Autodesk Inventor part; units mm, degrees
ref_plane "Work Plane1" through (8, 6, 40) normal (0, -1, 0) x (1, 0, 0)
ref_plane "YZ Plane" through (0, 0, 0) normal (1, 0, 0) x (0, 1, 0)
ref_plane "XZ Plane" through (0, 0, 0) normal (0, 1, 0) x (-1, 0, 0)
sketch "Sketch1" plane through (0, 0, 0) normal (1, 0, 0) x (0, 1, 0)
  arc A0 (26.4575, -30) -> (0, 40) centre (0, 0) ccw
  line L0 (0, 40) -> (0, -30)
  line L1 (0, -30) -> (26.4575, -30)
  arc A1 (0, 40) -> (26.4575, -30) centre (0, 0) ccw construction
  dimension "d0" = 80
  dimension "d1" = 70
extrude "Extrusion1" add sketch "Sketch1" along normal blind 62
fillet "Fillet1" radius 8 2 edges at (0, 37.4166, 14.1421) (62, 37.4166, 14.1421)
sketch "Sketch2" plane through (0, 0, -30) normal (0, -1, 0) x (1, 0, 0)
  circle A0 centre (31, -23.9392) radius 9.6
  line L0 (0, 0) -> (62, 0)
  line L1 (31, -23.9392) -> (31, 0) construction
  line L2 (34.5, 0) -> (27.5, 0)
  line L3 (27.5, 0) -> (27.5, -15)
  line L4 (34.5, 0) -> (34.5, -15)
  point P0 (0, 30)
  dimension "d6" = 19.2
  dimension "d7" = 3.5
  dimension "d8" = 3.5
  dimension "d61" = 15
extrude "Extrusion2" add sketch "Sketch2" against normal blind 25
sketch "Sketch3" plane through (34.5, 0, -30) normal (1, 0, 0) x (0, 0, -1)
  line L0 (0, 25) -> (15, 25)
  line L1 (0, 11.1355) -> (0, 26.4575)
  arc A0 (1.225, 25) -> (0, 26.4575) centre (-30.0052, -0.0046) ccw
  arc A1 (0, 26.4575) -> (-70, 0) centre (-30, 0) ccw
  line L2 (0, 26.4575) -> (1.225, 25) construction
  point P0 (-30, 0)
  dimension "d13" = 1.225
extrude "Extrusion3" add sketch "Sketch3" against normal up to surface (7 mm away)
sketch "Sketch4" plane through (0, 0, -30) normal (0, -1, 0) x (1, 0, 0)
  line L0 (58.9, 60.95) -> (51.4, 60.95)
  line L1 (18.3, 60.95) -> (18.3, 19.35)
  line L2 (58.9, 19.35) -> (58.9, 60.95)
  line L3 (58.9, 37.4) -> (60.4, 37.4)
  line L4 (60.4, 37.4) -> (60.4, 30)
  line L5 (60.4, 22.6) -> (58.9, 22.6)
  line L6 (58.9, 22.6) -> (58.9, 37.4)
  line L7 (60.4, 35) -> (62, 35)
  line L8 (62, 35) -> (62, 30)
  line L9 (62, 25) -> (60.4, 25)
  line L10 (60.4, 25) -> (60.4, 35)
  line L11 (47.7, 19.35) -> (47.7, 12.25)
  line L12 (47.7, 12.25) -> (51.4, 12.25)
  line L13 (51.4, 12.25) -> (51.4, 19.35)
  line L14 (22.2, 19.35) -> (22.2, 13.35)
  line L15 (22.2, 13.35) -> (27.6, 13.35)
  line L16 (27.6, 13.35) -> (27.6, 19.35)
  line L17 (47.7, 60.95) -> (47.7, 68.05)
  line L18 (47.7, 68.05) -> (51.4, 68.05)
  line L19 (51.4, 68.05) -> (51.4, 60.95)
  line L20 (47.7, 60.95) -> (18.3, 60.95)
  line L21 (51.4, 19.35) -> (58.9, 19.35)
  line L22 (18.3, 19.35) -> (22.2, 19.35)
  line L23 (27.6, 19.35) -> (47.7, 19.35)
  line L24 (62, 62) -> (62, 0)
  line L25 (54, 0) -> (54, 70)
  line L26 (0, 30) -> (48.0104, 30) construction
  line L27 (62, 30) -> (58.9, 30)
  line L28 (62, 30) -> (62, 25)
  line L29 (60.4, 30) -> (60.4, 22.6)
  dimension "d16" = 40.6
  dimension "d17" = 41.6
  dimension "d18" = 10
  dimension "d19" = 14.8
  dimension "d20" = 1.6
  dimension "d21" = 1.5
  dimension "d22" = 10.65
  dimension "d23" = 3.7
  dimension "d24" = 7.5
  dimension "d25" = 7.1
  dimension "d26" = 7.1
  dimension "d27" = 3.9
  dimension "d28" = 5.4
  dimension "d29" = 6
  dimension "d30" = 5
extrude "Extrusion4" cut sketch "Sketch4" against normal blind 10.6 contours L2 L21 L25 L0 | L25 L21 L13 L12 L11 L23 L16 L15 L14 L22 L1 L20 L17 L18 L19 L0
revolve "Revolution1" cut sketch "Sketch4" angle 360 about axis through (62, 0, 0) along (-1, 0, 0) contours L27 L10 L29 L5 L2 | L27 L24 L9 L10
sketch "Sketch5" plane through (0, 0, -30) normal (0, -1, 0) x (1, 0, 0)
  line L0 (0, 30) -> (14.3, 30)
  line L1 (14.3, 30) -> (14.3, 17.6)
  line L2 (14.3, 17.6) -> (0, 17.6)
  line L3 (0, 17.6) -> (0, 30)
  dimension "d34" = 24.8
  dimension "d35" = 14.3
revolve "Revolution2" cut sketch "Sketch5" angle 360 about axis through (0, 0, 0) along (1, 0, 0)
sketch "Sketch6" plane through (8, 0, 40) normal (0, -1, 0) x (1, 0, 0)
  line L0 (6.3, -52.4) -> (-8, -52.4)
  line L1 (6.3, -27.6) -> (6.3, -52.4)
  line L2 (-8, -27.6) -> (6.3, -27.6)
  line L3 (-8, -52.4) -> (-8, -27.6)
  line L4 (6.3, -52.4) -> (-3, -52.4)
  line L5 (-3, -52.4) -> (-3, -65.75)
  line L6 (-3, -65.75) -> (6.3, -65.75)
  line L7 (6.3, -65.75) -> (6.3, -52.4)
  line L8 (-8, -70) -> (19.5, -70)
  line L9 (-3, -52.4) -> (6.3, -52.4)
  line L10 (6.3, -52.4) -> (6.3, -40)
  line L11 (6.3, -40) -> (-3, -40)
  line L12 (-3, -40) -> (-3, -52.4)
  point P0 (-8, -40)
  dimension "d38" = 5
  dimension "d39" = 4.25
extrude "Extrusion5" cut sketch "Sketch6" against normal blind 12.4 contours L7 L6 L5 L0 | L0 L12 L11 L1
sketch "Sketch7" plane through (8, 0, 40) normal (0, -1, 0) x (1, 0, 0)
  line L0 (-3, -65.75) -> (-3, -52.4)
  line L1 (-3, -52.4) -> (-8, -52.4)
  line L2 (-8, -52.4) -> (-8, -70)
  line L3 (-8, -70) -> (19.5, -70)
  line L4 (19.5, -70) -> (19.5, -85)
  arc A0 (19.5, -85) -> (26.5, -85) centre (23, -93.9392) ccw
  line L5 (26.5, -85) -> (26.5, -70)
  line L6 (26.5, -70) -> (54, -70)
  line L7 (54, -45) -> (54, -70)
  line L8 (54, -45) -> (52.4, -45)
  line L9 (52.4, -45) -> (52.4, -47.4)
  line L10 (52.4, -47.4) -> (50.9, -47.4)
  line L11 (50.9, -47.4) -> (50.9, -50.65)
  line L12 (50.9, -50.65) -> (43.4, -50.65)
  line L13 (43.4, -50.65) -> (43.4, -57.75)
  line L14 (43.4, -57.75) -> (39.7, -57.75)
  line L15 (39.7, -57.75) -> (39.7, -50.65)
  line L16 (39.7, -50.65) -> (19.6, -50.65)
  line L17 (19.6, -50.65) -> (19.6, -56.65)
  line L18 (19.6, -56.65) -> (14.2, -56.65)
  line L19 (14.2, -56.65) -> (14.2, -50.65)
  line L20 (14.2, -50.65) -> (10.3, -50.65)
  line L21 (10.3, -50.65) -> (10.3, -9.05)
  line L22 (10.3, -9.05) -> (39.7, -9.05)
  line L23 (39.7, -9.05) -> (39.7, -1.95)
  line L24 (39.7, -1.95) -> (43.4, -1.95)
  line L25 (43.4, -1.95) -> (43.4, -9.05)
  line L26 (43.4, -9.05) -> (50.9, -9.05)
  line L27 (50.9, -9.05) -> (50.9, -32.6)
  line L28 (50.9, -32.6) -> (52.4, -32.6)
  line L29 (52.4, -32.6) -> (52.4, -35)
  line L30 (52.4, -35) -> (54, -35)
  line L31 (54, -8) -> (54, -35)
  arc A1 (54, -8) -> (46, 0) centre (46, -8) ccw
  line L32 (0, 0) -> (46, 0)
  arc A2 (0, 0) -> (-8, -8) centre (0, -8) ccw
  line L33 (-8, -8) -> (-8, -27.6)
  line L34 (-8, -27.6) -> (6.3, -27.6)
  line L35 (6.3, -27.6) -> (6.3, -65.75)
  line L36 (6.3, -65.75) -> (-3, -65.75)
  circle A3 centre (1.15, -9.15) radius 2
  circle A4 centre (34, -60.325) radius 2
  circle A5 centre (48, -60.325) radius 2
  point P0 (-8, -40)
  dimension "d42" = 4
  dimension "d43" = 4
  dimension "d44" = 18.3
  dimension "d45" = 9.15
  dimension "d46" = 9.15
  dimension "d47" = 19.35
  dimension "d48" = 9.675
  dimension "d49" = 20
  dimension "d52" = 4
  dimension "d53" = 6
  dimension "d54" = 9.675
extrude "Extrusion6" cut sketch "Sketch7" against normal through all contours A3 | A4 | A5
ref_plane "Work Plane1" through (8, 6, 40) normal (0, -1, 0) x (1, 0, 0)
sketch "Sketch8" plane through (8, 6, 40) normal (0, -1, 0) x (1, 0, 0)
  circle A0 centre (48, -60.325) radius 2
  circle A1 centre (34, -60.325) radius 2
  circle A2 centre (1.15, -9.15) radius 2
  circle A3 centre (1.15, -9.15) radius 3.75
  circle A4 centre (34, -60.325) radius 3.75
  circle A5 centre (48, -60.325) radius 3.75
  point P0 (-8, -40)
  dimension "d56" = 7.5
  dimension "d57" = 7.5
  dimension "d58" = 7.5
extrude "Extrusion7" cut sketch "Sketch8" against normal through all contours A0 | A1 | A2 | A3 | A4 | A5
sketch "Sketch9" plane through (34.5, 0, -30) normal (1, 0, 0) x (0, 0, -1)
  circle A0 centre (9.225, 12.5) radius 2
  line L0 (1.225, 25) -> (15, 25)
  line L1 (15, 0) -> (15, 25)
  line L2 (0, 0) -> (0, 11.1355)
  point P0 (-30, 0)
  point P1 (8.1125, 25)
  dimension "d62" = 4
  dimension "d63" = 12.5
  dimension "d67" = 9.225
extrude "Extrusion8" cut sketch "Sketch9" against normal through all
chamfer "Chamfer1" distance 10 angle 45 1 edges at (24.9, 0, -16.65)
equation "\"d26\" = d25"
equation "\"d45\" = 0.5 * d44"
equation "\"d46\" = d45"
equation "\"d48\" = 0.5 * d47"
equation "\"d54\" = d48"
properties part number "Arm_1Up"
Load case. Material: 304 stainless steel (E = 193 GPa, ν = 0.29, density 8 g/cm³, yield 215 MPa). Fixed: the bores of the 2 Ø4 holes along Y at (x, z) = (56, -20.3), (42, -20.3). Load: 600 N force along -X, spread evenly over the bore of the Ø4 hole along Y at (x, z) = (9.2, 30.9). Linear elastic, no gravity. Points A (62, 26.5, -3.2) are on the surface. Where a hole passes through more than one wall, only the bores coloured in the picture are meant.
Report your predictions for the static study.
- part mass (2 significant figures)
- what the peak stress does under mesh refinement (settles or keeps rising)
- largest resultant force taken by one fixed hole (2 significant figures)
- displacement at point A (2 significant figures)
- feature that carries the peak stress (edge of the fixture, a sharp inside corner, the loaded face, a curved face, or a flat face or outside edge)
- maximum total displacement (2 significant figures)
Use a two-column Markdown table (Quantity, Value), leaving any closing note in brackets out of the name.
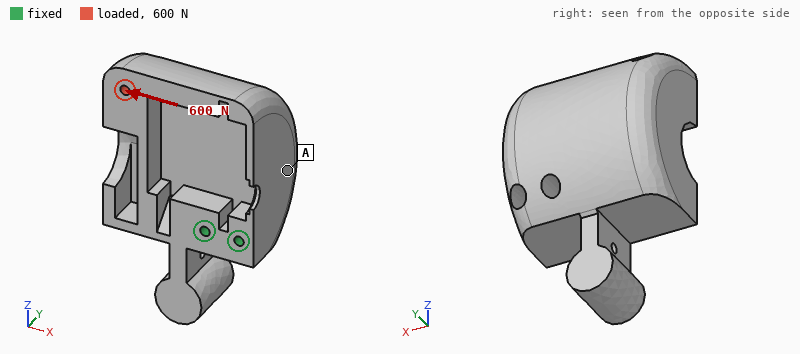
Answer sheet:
| Quantity | Value |
|---|---|
| part mass | 990 g |
| what the peak stress does under mesh refinement | keeps rising |
| largest resultant force taken by one fixed hole | 1.8 kN |
| displacement at point A | 5.3 µm |
| feature that carries the peak stress | edge of the fixture |
| maximum total displacement | 19 µm |
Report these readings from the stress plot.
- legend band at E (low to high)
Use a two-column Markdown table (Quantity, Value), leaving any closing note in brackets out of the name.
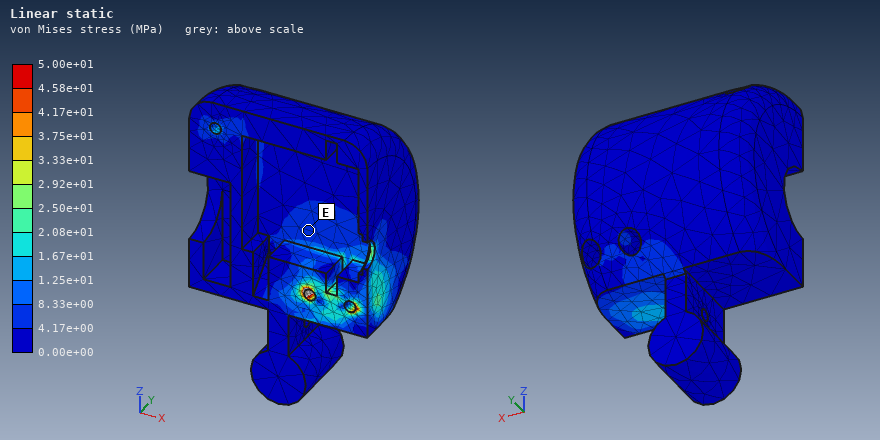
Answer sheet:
| Quantity | Value |
|---|---|
| legend band at E | 4.17e+00 to 8.33e+00 MPa |
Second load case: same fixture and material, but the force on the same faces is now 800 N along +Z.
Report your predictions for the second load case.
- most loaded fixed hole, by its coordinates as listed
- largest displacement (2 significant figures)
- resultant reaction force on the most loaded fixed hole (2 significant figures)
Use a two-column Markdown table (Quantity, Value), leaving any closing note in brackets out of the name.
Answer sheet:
| Quantity | Value |
|---|---|
| most loaded fixed hole, by its coordinates as listed | (42, -20.3) |
| largest displacement | 18 µm |
| resultant reaction force on the most loaded fixed hole | 2.2 kN |
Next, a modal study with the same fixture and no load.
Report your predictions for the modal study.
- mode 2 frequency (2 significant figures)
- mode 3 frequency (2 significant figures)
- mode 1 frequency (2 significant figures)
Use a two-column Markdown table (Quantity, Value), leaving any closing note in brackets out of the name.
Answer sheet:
| Quantity | Value |
|---|---|
| mode 2 frequency | 1500 Hz |
| mode 3 frequency | 2300 Hz |
| mode 1 frequency | 940 Hz |
